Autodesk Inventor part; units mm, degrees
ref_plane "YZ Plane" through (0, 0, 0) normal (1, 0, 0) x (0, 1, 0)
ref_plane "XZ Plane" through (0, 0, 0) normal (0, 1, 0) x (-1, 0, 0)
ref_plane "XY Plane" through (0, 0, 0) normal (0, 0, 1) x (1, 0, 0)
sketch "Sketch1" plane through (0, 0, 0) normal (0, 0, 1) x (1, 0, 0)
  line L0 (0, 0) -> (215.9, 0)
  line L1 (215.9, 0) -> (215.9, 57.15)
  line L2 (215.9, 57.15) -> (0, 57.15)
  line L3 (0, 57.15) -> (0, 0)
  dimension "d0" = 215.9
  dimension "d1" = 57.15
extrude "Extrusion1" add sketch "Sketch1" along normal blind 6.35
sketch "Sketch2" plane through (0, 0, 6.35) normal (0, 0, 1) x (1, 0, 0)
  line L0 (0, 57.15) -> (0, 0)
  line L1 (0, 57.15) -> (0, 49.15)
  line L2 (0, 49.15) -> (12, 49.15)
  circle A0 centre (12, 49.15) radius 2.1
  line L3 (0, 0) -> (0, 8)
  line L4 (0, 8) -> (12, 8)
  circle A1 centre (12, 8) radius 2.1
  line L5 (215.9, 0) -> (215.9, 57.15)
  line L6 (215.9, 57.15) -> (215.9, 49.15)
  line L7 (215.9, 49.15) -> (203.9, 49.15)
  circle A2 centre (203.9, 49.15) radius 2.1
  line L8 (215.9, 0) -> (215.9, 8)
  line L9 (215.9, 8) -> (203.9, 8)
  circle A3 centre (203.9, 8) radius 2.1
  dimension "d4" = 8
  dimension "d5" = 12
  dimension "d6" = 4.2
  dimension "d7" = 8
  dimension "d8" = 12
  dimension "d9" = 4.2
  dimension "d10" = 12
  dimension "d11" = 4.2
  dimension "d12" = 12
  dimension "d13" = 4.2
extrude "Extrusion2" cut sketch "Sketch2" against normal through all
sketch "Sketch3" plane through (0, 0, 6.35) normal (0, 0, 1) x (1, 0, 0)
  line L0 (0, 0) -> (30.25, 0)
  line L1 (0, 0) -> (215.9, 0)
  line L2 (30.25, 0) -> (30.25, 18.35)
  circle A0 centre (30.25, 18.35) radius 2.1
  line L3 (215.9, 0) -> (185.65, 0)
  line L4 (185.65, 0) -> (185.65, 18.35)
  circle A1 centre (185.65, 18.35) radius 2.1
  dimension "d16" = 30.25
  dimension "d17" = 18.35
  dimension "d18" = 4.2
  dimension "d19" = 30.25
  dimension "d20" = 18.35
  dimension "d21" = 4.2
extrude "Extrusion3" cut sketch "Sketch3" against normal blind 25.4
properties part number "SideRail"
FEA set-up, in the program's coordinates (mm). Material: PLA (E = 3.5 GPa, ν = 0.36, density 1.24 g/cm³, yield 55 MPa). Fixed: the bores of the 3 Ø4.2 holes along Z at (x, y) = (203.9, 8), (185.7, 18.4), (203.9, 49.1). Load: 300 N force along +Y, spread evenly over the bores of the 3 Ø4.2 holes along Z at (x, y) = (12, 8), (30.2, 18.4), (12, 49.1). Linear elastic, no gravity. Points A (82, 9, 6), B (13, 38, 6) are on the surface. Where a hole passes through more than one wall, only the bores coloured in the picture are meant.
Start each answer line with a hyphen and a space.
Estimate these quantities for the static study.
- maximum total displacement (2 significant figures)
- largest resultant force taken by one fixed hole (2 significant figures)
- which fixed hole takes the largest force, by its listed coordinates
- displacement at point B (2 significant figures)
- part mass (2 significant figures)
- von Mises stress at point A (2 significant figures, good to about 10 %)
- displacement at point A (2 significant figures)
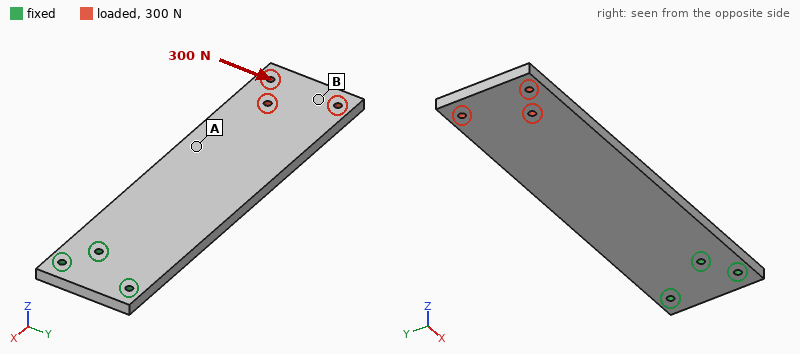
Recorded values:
- 2.2 mm
- 1.2 kN
- (203.9, 49.1)
- 2.0 mm
- 97 g
- 3.9 MPa
- 1.0 mm
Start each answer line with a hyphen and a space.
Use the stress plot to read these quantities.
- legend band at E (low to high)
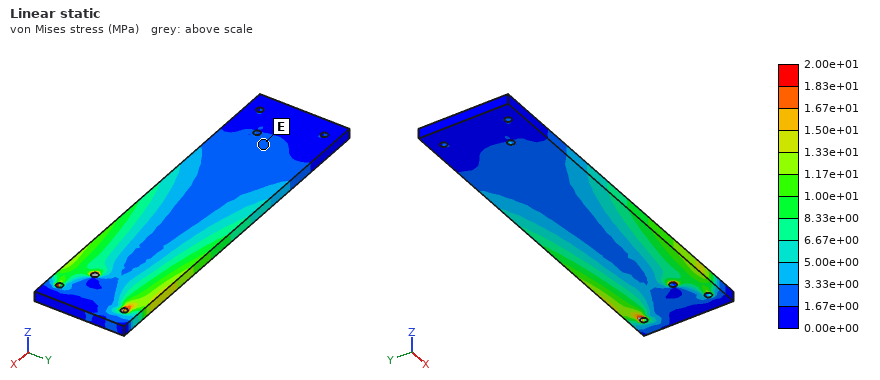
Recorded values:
- 1.67e+00 to 3.33e+00 MPa
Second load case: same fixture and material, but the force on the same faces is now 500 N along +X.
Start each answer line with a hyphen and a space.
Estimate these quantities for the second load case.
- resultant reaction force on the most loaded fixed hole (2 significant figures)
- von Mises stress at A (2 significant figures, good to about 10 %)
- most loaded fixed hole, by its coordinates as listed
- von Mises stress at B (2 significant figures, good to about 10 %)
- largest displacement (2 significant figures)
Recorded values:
- 260 N
- 1.7 MPa
- (185.7, 18.4)
- 0.57 MPa
- 0.12 mm
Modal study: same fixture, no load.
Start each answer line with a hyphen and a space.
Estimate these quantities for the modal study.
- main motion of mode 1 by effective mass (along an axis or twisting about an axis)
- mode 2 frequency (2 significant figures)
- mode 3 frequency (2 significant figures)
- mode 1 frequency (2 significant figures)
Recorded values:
- along Z
- 290 Hz
- 310 Hz
- 49 Hz
